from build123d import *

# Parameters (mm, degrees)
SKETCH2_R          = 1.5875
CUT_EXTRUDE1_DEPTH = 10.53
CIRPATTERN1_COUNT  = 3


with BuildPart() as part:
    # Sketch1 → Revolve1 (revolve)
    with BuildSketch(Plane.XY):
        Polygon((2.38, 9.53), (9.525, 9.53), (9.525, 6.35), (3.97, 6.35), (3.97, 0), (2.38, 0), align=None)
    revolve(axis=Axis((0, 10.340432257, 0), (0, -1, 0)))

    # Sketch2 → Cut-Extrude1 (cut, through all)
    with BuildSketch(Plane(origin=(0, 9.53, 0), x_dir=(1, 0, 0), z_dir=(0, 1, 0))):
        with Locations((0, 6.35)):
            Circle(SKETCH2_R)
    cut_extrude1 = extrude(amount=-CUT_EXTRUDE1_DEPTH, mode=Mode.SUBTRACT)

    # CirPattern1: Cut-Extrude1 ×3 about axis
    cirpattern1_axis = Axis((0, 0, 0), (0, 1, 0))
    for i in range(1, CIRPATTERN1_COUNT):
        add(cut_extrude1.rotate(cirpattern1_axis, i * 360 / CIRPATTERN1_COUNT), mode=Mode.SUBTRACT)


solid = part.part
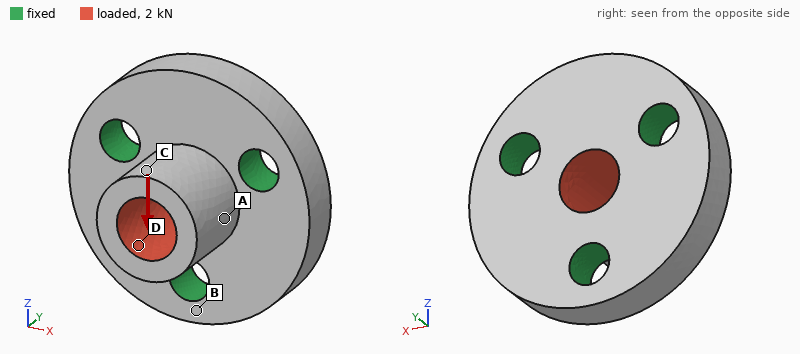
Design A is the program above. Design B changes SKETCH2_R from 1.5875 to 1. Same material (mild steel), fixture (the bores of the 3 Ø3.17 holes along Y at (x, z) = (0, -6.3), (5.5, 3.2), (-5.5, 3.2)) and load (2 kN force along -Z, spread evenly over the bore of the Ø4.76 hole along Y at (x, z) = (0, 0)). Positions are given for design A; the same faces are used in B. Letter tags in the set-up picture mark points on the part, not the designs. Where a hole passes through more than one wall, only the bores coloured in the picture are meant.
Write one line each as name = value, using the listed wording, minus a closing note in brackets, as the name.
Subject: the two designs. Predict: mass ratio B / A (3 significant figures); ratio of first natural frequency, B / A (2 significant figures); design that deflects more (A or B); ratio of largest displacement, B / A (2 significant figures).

mass ratio B / A = 1.05
ratio of first natural frequency, B / A = 0.87
design that deflects more = B
ratio of largest displacement, B / A = 1.1
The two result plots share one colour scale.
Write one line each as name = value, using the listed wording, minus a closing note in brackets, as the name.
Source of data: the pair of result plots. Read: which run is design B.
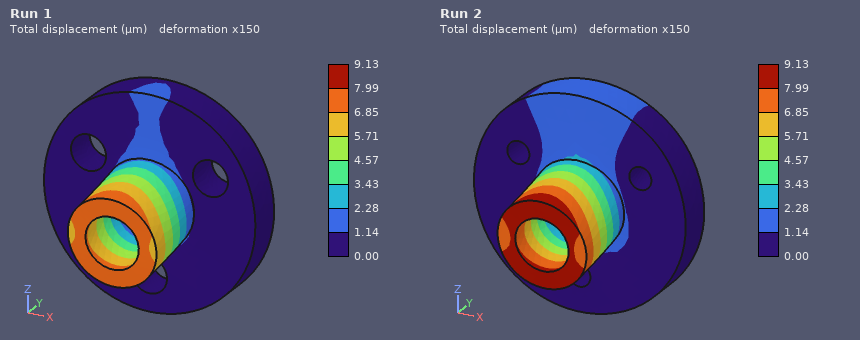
which run is design B = Run 2
